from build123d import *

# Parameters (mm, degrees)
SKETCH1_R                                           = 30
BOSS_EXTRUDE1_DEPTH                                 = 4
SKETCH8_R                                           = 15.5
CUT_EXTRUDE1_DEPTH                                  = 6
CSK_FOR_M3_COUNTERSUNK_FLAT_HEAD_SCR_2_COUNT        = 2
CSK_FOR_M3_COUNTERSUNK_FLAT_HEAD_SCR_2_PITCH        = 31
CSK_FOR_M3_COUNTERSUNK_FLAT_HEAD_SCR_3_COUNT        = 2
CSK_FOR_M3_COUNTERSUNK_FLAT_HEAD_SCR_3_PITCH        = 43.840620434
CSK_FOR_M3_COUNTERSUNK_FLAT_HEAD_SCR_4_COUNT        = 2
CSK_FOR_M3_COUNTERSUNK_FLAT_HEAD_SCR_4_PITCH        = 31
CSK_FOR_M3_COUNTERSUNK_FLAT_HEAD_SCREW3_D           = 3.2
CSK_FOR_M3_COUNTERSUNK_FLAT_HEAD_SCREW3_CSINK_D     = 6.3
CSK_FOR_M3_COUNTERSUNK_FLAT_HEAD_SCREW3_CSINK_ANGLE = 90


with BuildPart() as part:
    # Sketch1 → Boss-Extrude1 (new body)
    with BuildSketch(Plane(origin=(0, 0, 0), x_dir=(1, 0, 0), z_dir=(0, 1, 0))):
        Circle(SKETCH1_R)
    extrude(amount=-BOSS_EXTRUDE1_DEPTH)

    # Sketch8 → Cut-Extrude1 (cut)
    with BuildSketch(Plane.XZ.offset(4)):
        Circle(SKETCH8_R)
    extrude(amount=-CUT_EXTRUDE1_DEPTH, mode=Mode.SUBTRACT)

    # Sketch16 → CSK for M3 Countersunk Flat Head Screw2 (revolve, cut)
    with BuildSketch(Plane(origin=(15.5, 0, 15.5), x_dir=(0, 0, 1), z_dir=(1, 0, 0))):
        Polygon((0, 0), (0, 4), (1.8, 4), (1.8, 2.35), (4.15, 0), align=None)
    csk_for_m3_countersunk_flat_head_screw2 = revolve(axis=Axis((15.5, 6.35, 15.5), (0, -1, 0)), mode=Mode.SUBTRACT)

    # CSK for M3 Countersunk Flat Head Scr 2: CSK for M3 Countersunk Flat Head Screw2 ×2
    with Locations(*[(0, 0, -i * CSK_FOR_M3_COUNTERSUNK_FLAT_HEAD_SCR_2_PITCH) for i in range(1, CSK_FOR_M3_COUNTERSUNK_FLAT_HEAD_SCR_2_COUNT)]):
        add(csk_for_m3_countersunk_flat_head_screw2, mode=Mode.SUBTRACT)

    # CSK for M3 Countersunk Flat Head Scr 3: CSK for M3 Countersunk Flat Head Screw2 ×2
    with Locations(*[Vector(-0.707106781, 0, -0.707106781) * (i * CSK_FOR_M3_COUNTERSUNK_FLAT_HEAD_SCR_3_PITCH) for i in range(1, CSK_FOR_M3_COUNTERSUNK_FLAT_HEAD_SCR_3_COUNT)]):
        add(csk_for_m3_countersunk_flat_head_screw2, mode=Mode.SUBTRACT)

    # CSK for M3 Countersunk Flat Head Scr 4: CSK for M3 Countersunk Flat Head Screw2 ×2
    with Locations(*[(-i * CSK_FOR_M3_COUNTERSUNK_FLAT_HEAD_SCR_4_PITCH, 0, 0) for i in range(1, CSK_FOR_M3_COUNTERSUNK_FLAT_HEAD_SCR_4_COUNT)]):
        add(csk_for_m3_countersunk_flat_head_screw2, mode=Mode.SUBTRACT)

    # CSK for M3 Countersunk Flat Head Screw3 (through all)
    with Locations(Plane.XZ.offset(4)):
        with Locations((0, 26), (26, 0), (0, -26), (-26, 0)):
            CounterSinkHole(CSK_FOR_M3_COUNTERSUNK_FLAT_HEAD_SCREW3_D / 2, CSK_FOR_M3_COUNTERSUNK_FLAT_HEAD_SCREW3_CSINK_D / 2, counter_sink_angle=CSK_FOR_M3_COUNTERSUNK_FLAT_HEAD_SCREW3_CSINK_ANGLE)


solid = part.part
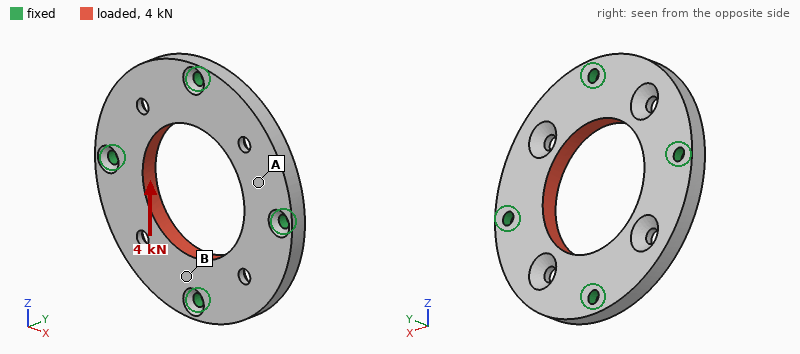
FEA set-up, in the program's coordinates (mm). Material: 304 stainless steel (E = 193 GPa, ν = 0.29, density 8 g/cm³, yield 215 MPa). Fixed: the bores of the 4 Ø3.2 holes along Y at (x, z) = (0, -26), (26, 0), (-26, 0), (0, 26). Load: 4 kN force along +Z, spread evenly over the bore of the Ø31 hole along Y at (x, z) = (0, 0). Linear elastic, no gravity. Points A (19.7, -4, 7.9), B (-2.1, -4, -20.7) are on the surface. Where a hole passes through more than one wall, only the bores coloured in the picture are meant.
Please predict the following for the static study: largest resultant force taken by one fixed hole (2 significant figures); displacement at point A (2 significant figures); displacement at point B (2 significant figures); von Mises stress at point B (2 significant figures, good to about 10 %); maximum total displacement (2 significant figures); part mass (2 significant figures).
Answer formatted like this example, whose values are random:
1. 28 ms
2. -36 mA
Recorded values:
1. 1.0 kN
2. 2.0 µm
3. 1.2 µm
4. 22 MPa
5. 2.8 µm
6. 62 g
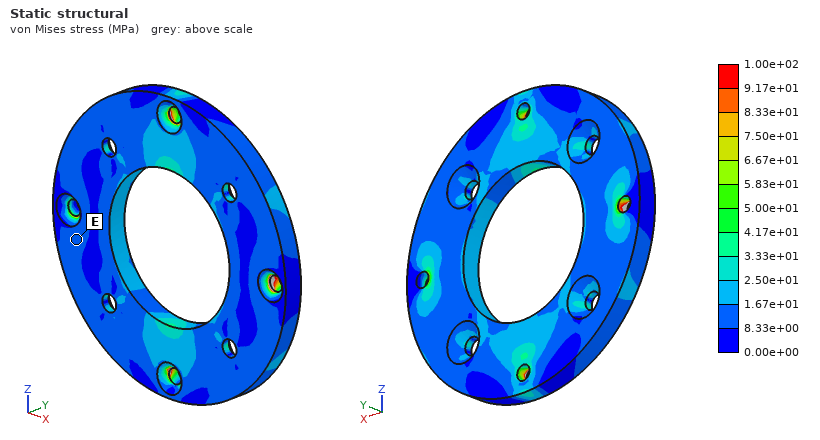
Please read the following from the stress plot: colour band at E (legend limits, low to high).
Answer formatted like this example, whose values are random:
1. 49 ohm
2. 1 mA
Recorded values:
1. 8.33e+00 to 1.67e+01 MPa
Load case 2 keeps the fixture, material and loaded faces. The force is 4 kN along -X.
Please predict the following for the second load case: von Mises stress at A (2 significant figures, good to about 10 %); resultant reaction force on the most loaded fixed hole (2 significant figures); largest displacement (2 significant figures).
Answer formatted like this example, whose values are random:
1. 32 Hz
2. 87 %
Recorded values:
1. 15 MPa
2. 1.0 kN
3. 2.8 µm
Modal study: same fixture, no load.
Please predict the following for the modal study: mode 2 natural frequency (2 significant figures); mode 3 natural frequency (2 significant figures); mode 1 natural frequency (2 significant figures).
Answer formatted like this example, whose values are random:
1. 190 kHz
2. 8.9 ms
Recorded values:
1. 10 kHz
2. 10 kHz
3. 9000 Hz
